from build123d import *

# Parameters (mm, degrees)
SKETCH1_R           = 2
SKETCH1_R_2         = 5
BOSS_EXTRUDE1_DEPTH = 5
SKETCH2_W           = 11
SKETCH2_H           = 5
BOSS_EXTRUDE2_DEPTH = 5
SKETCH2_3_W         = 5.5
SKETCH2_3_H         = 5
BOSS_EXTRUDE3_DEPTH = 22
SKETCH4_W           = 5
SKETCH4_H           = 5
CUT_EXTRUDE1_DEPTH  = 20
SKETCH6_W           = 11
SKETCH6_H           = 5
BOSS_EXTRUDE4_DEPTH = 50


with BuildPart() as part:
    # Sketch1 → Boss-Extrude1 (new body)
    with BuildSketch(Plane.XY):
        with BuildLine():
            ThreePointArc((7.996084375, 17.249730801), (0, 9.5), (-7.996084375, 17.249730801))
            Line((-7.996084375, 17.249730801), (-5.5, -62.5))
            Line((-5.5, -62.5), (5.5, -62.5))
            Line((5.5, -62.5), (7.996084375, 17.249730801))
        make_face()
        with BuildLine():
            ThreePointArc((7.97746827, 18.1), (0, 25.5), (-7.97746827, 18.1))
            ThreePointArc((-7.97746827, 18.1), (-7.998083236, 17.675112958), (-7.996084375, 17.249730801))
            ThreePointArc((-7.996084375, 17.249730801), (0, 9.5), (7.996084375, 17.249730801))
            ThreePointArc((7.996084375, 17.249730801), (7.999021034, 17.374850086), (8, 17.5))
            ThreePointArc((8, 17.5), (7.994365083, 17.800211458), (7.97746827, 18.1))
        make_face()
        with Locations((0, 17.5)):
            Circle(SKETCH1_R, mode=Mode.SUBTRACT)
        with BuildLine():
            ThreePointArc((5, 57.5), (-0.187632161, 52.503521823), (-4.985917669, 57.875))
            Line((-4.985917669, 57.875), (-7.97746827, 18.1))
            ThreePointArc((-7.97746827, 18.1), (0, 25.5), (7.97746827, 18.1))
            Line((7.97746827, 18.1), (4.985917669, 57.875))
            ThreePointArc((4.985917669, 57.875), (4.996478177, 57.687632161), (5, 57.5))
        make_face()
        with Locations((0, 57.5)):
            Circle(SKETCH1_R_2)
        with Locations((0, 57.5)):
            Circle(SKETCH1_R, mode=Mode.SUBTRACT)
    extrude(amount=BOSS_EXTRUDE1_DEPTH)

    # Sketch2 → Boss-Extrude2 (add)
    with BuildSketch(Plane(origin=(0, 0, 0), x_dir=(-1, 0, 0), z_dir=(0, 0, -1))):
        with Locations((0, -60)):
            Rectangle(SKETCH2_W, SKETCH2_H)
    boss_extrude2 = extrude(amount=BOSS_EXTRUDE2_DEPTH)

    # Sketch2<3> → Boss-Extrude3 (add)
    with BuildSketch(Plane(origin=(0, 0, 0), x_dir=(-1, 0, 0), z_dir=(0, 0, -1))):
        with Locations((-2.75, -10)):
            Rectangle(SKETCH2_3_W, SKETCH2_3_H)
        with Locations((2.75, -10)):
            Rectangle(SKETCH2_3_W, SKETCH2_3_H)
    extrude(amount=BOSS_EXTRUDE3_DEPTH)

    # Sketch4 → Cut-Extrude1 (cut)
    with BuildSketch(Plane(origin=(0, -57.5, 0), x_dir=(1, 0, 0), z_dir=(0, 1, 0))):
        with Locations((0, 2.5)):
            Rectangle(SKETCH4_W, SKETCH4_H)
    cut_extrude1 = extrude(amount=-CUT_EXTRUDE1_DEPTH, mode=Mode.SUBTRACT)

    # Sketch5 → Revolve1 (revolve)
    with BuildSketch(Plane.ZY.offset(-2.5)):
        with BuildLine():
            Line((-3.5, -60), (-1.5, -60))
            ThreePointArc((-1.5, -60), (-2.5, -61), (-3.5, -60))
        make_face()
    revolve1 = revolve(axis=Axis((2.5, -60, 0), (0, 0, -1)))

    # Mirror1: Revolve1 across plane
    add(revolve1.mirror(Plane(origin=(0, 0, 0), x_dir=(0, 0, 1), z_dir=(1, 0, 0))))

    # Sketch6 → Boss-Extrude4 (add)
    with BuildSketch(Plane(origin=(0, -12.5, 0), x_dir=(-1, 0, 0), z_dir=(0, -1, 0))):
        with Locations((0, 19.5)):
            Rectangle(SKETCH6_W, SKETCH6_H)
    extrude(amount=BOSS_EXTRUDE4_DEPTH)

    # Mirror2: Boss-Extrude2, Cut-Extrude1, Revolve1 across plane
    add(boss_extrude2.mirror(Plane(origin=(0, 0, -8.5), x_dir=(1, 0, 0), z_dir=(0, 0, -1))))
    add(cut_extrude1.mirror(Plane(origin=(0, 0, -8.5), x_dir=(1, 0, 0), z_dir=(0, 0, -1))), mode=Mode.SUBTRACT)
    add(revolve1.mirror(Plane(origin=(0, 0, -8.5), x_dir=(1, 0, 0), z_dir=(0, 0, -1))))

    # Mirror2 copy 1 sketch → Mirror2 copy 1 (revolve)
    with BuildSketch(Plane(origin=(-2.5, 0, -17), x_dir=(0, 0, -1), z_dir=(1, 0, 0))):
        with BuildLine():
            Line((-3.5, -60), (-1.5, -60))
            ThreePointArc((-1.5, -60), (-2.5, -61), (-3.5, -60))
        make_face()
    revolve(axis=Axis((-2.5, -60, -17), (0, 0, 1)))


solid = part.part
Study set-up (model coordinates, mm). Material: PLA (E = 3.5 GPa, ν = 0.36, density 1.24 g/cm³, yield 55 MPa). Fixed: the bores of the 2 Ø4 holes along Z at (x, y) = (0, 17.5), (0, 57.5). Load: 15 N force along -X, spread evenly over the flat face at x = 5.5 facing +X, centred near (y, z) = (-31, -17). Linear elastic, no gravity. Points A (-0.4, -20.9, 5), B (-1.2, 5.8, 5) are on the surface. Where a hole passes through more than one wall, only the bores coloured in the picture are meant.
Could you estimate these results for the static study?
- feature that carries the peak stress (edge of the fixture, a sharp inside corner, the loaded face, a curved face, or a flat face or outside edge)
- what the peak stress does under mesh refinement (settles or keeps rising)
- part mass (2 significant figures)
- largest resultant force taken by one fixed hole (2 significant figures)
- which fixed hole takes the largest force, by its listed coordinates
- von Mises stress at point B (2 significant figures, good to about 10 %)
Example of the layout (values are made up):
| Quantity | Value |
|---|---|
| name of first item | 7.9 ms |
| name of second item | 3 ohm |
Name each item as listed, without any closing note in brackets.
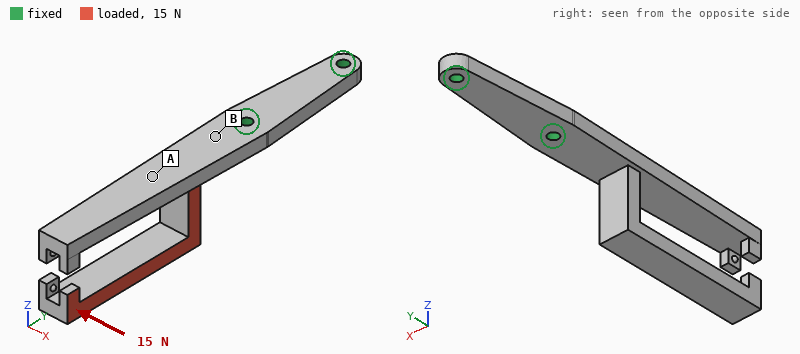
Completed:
| Quantity | Value |
|---|---|
| feature that carries the peak stress | edge of the fixture |
| what the peak stress does under mesh refinement | keeps rising |
| part mass | 15 g |
| largest resultant force taken by one fixed hole | 25 N |
| which fixed hole takes the largest force, by its listed coordinates | (0, 17.5) |
| von Mises stress at point B | 4.1 MPa |
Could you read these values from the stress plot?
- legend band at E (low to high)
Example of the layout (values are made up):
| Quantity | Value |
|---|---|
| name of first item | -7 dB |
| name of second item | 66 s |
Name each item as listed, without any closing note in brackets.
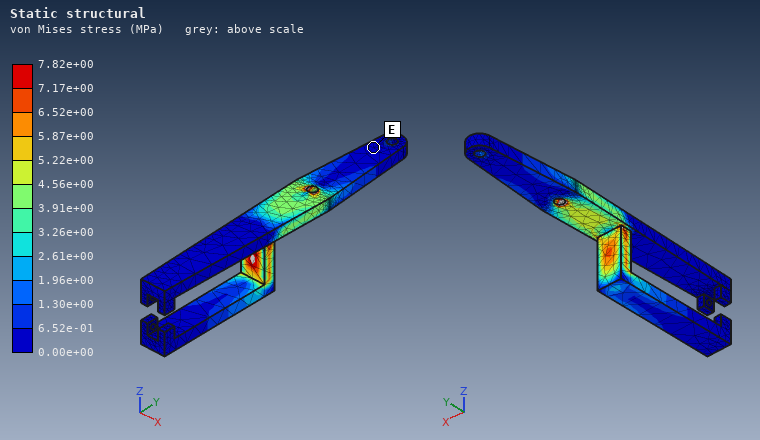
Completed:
| Quantity | Value |
|---|---|
| legend band at E | 0.00e+00 to 6.52e-01 MPa |
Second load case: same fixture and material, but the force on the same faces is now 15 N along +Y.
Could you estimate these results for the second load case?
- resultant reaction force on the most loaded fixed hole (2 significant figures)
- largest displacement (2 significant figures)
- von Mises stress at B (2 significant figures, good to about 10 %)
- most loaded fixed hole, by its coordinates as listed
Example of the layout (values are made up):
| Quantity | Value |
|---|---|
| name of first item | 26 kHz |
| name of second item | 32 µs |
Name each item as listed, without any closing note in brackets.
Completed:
| Quantity | Value |
|---|---|
| resultant reaction force on the most loaded fixed hole | 14 N |
| largest displacement | 1.3 mm |
| von Mises stress at B | 4.2 MPa |
| most loaded fixed hole, by its coordinates as listed | (0, 17.5) |
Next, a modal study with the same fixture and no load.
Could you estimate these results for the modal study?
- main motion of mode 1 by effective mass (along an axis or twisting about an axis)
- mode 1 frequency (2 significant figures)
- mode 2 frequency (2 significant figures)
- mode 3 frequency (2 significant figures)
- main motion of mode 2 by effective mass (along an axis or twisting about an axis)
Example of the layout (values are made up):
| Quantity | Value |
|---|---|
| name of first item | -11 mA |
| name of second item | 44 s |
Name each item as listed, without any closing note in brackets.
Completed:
| Quantity | Value |
|---|---|
| main motion of mode 1 by effective mass | along Z |
| mode 1 frequency | 150 Hz |
| mode 2 frequency | 290 Hz |
| mode 3 frequency | 360 Hz |
| main motion of mode 2 by effective mass | along X |
